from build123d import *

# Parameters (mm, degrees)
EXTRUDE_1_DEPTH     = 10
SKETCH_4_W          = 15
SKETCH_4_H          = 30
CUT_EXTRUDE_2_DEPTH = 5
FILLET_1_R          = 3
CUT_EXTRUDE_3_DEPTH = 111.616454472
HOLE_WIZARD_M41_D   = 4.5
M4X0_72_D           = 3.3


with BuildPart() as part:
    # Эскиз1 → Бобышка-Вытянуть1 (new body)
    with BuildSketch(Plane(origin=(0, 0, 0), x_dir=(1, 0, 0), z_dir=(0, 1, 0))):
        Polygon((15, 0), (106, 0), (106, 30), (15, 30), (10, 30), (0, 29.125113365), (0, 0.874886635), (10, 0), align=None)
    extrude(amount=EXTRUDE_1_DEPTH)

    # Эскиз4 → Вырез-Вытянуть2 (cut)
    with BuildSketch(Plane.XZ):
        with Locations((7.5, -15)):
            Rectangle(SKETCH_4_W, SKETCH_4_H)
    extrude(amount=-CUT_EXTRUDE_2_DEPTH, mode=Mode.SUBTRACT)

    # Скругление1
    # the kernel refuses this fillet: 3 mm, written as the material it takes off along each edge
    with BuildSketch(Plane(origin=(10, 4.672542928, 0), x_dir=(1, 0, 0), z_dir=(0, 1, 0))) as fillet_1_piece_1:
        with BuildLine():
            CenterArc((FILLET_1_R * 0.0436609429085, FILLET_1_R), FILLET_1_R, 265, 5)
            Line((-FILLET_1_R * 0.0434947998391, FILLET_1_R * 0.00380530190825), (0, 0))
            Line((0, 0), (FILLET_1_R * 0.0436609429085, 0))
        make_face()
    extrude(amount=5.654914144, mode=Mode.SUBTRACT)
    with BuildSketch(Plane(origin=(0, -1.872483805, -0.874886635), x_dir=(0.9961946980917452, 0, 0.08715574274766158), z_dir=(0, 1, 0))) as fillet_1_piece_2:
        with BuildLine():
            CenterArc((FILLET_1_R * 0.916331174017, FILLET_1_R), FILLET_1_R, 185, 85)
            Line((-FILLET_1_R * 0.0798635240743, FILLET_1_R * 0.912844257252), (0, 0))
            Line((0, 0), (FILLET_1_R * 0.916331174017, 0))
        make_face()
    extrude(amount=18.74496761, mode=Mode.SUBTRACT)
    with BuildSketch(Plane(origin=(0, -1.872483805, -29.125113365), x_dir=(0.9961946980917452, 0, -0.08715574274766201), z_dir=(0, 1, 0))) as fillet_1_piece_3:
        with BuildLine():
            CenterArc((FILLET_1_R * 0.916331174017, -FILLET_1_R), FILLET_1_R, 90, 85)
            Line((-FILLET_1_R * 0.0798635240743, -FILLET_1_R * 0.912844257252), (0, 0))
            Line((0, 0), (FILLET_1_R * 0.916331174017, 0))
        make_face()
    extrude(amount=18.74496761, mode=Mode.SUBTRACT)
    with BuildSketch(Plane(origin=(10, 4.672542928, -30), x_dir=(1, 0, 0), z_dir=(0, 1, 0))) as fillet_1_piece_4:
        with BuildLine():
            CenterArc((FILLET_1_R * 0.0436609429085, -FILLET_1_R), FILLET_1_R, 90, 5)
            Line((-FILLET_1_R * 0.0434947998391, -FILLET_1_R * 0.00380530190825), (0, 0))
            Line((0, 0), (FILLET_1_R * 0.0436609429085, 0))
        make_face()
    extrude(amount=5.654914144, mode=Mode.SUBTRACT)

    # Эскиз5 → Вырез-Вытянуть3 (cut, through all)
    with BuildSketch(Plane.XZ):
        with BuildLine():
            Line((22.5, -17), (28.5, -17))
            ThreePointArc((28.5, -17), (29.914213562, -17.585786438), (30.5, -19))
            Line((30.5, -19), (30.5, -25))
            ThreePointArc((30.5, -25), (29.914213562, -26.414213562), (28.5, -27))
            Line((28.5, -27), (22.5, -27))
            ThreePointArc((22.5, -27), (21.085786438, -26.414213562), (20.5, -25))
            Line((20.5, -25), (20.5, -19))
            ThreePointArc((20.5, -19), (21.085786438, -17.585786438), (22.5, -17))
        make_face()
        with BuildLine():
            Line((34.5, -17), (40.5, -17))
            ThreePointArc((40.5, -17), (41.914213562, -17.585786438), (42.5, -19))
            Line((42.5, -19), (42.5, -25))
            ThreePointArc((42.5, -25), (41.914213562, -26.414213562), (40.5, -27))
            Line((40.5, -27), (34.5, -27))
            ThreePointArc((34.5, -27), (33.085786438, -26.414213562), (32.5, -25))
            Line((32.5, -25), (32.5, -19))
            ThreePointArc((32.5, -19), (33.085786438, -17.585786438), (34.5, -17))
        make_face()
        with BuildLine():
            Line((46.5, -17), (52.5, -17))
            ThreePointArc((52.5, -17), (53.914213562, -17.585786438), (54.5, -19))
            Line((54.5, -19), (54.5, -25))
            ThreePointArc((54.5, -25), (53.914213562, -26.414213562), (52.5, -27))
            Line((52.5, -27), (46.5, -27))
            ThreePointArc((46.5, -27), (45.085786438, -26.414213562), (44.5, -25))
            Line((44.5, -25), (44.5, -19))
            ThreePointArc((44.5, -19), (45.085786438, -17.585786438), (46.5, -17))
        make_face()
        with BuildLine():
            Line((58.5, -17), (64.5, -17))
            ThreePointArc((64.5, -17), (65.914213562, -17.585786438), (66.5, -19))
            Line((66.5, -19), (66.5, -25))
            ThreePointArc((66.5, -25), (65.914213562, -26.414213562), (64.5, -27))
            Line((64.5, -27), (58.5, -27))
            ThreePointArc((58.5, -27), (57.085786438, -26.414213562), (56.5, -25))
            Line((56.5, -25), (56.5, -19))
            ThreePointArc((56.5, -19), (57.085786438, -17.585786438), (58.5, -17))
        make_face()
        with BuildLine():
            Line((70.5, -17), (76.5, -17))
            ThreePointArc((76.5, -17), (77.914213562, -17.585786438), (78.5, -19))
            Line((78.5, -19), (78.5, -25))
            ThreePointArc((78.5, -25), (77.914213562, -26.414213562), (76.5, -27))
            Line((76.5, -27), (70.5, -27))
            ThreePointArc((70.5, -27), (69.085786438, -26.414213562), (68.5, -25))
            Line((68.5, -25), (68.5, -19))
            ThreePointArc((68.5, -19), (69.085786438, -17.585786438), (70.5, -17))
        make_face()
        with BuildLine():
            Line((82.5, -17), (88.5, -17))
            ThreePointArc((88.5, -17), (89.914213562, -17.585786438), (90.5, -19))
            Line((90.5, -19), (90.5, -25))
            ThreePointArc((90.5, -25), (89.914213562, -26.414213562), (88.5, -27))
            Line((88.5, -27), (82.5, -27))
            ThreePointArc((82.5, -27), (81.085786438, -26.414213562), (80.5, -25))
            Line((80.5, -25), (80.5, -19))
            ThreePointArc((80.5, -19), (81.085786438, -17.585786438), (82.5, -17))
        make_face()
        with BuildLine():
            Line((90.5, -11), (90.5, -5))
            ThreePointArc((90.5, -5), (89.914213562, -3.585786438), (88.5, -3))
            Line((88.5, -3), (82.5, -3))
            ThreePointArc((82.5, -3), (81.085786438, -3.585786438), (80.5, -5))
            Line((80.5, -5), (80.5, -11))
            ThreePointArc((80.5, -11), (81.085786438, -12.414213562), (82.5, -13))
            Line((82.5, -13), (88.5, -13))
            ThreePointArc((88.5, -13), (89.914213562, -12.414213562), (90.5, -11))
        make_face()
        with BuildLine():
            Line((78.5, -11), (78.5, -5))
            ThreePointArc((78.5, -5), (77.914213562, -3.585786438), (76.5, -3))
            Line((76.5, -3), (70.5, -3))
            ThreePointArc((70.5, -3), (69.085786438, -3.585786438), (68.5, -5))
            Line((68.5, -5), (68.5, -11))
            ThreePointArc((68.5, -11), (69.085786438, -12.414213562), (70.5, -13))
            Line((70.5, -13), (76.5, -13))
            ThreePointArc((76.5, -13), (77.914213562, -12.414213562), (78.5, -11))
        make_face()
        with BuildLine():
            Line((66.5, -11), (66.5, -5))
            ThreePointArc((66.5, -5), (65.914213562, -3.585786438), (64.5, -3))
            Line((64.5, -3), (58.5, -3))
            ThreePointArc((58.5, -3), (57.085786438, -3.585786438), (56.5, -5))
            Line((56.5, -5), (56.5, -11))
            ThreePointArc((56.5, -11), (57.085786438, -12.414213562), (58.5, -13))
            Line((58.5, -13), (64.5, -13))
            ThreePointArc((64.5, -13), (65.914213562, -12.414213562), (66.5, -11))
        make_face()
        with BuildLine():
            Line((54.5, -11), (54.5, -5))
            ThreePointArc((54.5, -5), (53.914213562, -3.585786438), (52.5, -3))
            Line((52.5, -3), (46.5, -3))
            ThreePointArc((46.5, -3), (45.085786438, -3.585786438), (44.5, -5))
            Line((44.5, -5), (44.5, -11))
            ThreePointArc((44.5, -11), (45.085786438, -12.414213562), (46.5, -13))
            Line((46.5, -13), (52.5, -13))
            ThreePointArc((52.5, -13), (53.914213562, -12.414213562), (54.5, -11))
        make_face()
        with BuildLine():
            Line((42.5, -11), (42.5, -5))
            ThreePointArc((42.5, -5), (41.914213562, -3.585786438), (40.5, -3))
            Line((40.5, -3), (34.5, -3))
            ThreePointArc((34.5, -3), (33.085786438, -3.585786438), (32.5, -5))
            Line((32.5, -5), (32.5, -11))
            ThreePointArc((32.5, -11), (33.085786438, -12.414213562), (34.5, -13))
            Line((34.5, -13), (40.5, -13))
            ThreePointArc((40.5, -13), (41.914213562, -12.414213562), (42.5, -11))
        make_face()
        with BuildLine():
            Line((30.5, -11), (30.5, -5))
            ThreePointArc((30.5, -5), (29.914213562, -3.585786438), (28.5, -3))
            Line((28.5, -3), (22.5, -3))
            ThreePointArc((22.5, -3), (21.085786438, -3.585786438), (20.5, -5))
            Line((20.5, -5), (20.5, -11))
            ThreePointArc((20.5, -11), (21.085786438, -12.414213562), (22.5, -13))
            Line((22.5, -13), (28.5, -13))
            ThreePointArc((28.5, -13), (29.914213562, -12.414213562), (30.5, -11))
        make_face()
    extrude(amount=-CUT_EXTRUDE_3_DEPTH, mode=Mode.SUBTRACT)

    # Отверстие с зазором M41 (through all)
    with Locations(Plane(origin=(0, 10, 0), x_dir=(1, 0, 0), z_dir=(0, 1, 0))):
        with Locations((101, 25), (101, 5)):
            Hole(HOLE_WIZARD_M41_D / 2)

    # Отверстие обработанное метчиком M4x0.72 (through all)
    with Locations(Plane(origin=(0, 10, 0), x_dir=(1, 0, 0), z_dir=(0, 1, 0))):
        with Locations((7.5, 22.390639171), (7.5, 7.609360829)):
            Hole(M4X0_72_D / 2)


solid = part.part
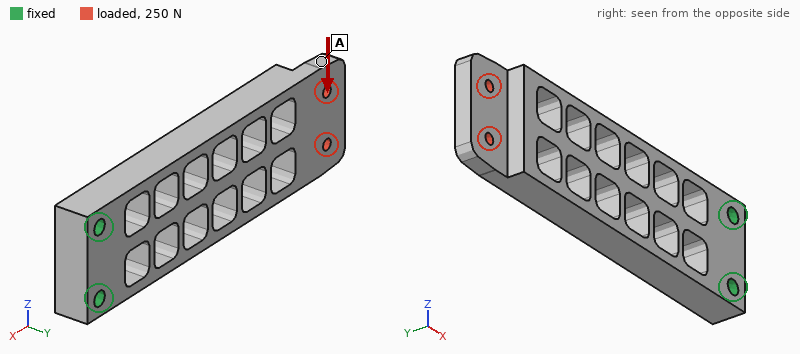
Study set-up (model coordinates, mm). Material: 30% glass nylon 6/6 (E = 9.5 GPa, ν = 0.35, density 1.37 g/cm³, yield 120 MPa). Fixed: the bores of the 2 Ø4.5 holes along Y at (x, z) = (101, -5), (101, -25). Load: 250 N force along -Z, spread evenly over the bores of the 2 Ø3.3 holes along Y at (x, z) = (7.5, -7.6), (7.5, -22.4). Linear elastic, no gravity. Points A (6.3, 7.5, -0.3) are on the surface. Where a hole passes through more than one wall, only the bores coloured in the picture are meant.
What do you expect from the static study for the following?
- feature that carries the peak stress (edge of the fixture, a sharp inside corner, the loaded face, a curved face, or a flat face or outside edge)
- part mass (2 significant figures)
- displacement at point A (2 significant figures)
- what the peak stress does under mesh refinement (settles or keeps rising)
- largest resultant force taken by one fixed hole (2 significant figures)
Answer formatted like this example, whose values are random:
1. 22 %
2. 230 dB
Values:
1. a sharp inside corner
2. 24 g
3. 1.2 mm
4. keeps rising
5. 1.0 kN
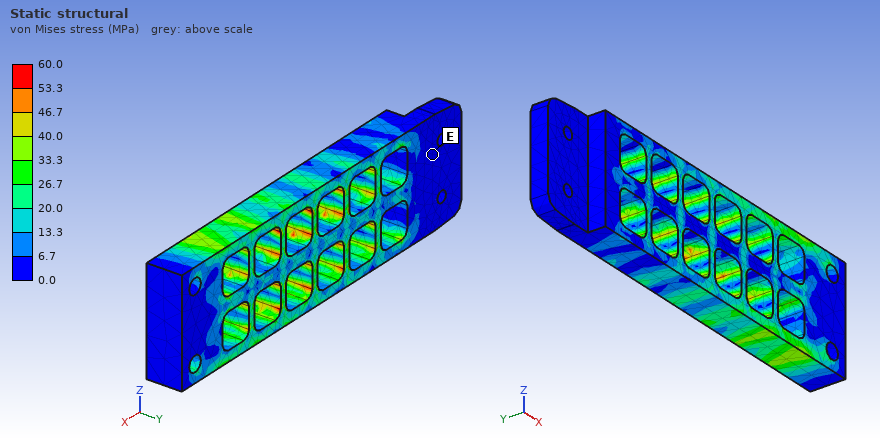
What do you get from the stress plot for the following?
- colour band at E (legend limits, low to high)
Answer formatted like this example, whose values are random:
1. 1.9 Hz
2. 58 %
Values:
1. 0.0 to 6.7 MPa
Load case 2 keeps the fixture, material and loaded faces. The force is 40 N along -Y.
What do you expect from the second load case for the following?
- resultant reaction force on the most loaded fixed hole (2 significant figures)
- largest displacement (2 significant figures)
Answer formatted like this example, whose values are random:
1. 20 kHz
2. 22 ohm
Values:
1. 20 N
2. 1.3 mm
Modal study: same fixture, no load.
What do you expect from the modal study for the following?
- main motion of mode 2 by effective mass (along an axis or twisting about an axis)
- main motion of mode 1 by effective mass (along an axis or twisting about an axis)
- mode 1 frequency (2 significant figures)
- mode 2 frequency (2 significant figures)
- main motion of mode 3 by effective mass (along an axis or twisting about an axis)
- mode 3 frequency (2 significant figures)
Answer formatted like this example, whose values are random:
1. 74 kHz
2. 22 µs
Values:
1. along Z
2. along Y
3. 370 Hz
4. 820 Hz
5. twisting about X
6. 1200 Hz
